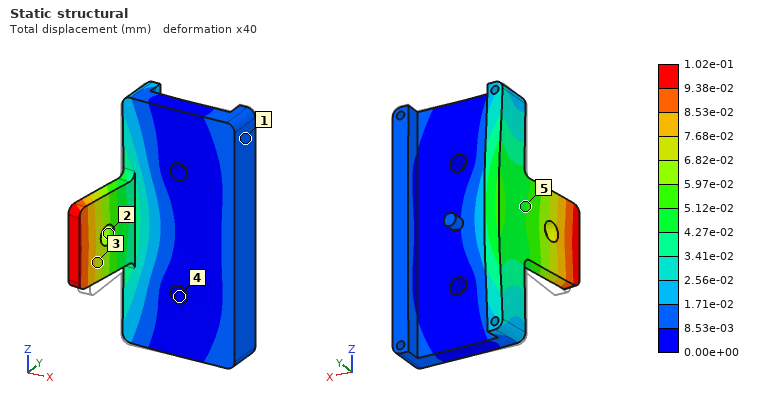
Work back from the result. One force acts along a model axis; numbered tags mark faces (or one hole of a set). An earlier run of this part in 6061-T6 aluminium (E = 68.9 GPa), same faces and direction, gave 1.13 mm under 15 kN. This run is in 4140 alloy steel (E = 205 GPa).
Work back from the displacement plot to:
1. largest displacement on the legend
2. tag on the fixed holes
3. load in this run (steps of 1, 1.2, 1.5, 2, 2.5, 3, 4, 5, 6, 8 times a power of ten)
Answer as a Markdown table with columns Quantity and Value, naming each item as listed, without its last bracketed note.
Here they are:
| Quantity | Value |
|---|---|
| largest displacement on the legend | 1.02e-01 mm |
| tag on the fixed holes | 4 |
| load in this run | 4 kN |
